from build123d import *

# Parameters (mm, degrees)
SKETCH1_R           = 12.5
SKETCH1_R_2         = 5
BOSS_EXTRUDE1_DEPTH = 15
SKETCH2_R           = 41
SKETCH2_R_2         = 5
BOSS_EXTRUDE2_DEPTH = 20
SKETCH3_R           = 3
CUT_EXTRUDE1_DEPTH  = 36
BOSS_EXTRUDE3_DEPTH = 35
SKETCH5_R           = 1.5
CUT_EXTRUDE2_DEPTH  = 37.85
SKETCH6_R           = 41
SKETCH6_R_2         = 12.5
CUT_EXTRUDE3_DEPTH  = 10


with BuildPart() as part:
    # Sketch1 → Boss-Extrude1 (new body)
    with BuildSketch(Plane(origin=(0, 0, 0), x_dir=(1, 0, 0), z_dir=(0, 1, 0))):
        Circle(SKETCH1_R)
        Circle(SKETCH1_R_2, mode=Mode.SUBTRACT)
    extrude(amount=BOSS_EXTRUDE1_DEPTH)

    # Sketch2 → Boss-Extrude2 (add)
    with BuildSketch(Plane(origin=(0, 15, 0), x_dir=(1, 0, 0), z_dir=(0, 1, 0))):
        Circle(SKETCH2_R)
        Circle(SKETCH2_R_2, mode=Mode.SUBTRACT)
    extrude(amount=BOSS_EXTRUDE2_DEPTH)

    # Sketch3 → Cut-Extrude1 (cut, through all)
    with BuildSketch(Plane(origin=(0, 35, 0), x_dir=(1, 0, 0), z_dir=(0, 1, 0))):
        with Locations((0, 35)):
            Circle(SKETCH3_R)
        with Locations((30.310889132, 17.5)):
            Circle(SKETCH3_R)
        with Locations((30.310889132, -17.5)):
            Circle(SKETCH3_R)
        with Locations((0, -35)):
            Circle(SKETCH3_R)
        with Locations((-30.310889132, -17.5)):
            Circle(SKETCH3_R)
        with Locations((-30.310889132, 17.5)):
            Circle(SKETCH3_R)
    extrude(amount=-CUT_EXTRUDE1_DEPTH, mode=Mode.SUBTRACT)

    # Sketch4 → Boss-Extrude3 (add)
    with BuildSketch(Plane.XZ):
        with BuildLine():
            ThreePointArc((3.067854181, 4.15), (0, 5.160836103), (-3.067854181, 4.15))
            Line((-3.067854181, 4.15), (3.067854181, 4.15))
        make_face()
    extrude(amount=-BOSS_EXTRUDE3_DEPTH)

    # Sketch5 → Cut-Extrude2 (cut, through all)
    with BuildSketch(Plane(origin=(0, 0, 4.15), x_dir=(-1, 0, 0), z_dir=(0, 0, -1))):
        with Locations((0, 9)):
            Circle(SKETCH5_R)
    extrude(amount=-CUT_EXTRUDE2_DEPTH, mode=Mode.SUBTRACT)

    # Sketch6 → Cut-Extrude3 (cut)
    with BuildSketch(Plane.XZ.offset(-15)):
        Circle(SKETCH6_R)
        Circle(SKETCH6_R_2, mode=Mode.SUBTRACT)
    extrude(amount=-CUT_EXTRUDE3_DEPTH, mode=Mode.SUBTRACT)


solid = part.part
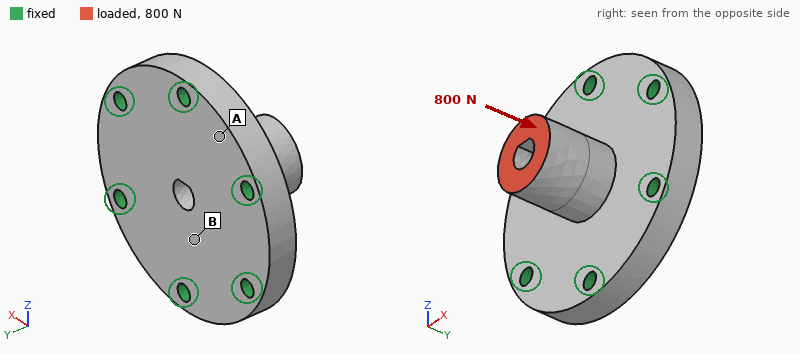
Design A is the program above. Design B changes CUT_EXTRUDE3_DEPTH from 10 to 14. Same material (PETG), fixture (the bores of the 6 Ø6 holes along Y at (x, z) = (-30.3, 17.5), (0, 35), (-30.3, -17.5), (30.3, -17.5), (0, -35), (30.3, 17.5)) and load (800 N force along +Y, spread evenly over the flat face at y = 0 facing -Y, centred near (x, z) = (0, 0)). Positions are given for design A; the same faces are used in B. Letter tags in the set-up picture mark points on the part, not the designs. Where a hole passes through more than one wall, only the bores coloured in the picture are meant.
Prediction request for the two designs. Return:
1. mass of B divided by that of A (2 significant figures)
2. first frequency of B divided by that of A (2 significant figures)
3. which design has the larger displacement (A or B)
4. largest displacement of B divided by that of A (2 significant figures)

0.70
0.60
B
2.6
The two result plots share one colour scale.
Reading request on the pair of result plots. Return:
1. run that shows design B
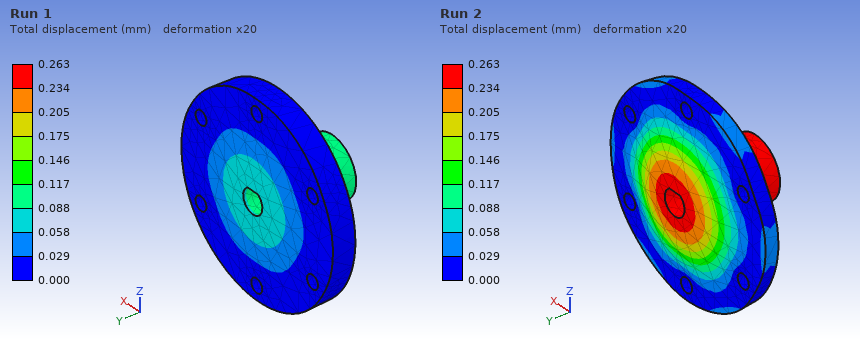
Run 2
